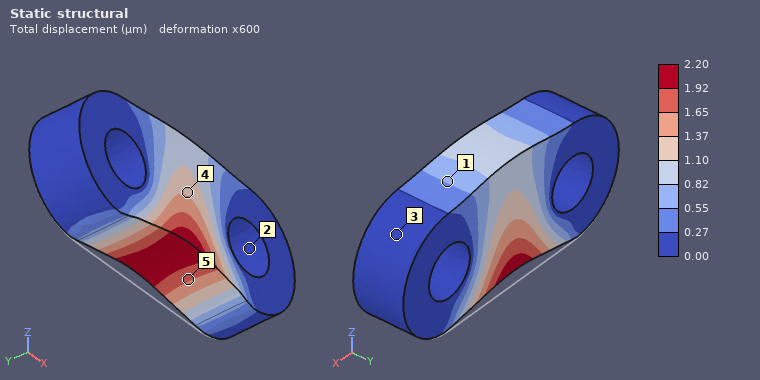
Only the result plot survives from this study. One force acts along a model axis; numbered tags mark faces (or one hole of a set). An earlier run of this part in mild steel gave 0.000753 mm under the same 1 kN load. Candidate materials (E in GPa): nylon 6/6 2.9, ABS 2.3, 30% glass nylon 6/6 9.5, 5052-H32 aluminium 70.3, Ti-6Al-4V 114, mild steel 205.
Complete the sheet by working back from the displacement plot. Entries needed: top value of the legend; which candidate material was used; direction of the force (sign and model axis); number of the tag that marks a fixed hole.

2.20 µm
5052-H32 aluminium
+Z
2
